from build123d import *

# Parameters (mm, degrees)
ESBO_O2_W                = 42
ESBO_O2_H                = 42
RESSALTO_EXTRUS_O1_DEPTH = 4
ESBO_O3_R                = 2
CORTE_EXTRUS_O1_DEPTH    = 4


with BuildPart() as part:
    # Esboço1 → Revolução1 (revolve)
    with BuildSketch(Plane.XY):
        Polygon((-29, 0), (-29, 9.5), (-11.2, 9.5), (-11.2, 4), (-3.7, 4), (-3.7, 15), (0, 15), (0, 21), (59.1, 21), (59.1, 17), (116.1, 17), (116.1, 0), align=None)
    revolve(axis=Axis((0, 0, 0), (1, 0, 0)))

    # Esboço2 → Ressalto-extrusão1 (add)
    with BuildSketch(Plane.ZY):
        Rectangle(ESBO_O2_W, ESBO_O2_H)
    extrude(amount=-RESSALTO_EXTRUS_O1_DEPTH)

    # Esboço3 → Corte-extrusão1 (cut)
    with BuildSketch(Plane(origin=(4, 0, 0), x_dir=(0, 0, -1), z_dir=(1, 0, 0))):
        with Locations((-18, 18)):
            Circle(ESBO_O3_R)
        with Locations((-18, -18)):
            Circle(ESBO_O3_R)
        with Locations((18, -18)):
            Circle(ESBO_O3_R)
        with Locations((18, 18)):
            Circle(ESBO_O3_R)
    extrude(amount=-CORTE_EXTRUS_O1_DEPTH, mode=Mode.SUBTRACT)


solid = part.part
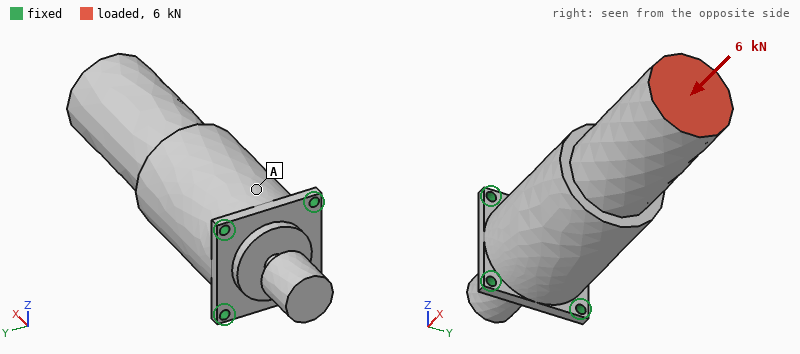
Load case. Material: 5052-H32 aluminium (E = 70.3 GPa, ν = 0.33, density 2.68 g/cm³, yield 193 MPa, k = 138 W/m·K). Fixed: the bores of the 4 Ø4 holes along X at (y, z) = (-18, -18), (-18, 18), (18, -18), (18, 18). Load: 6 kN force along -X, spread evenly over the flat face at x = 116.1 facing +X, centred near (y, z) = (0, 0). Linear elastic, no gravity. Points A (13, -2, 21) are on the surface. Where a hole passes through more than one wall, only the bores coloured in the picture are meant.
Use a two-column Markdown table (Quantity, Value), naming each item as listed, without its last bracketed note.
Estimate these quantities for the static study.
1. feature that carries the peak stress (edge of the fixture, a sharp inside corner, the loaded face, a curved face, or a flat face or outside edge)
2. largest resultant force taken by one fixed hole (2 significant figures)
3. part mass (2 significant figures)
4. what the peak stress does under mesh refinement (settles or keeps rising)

| Quantity | Value |
|---|---|
| feature that carries the peak stress | edge of the fixture |
| largest resultant force taken by one fixed hole | 1.6 kN |
| part mass | 380 g |
| what the peak stress does under mesh refinement | keeps rising |
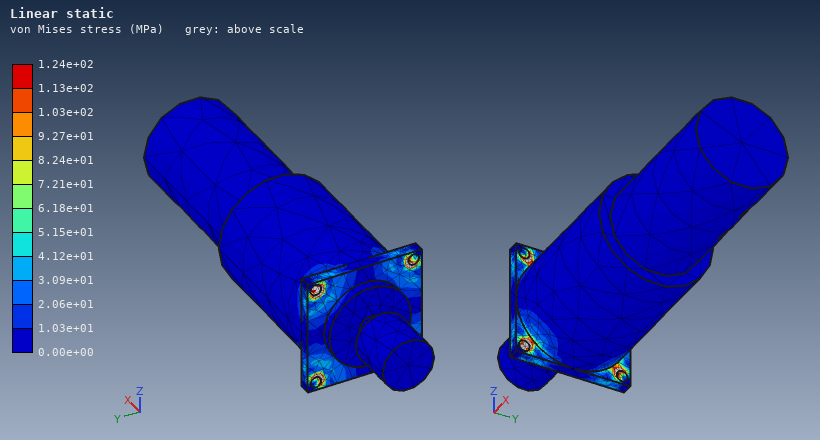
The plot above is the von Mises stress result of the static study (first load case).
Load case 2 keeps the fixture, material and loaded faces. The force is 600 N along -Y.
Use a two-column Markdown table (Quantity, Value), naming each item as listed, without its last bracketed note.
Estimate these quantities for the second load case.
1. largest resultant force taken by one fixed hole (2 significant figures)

| Quantity | Value |
|---|---|
| largest resultant force taken by one fixed hole | 1.1 kN |
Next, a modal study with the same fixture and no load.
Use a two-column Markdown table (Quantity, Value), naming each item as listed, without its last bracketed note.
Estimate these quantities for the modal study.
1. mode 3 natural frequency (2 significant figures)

| Quantity | Value |
|---|---|
| mode 3 natural frequency | 3300 Hz |
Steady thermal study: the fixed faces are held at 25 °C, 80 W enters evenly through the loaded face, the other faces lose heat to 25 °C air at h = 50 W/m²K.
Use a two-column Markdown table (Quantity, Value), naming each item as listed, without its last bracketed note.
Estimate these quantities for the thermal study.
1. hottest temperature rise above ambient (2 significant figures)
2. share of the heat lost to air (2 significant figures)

| Quantity | Value |
|---|---|
| hottest temperature rise above ambient | 65 K |
| share of the heat lost to air | 32 % |
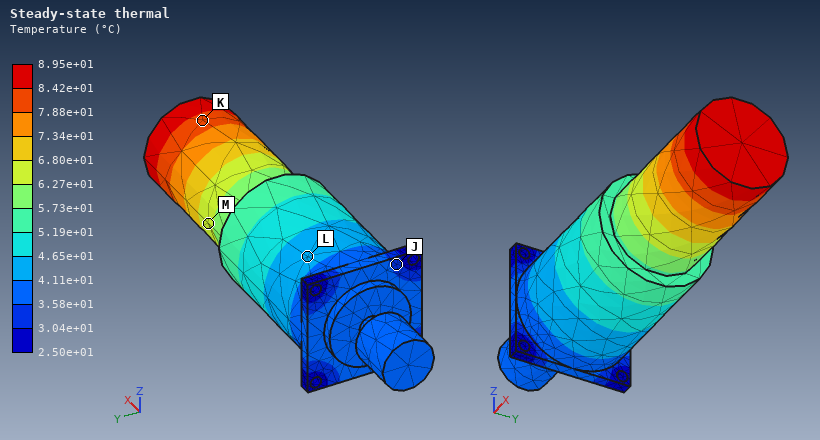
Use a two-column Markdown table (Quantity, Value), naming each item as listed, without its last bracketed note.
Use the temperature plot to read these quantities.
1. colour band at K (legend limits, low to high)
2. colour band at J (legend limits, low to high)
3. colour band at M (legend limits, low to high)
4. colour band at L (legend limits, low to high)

| Quantity | Value |
|---|---|
| colour band at K | 7.88e+01 to 8.42e+01 °C |
| colour band at J | 3.04e+01 to 3.58e+01 °C |
| colour band at M | 6.27e+01 to 6.80e+01 °C |
| colour band at L | 4.11e+01 to 4.65e+01 °C |
